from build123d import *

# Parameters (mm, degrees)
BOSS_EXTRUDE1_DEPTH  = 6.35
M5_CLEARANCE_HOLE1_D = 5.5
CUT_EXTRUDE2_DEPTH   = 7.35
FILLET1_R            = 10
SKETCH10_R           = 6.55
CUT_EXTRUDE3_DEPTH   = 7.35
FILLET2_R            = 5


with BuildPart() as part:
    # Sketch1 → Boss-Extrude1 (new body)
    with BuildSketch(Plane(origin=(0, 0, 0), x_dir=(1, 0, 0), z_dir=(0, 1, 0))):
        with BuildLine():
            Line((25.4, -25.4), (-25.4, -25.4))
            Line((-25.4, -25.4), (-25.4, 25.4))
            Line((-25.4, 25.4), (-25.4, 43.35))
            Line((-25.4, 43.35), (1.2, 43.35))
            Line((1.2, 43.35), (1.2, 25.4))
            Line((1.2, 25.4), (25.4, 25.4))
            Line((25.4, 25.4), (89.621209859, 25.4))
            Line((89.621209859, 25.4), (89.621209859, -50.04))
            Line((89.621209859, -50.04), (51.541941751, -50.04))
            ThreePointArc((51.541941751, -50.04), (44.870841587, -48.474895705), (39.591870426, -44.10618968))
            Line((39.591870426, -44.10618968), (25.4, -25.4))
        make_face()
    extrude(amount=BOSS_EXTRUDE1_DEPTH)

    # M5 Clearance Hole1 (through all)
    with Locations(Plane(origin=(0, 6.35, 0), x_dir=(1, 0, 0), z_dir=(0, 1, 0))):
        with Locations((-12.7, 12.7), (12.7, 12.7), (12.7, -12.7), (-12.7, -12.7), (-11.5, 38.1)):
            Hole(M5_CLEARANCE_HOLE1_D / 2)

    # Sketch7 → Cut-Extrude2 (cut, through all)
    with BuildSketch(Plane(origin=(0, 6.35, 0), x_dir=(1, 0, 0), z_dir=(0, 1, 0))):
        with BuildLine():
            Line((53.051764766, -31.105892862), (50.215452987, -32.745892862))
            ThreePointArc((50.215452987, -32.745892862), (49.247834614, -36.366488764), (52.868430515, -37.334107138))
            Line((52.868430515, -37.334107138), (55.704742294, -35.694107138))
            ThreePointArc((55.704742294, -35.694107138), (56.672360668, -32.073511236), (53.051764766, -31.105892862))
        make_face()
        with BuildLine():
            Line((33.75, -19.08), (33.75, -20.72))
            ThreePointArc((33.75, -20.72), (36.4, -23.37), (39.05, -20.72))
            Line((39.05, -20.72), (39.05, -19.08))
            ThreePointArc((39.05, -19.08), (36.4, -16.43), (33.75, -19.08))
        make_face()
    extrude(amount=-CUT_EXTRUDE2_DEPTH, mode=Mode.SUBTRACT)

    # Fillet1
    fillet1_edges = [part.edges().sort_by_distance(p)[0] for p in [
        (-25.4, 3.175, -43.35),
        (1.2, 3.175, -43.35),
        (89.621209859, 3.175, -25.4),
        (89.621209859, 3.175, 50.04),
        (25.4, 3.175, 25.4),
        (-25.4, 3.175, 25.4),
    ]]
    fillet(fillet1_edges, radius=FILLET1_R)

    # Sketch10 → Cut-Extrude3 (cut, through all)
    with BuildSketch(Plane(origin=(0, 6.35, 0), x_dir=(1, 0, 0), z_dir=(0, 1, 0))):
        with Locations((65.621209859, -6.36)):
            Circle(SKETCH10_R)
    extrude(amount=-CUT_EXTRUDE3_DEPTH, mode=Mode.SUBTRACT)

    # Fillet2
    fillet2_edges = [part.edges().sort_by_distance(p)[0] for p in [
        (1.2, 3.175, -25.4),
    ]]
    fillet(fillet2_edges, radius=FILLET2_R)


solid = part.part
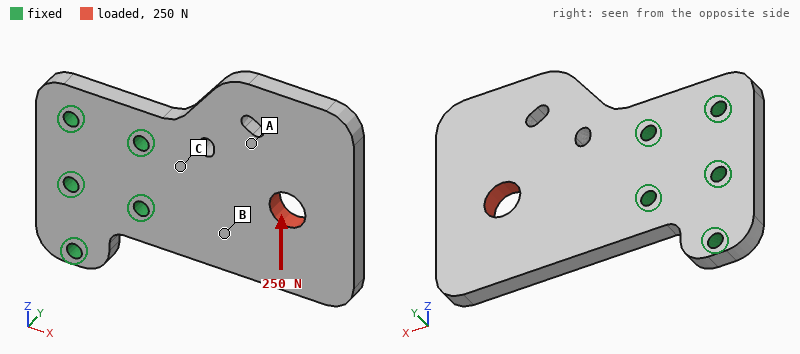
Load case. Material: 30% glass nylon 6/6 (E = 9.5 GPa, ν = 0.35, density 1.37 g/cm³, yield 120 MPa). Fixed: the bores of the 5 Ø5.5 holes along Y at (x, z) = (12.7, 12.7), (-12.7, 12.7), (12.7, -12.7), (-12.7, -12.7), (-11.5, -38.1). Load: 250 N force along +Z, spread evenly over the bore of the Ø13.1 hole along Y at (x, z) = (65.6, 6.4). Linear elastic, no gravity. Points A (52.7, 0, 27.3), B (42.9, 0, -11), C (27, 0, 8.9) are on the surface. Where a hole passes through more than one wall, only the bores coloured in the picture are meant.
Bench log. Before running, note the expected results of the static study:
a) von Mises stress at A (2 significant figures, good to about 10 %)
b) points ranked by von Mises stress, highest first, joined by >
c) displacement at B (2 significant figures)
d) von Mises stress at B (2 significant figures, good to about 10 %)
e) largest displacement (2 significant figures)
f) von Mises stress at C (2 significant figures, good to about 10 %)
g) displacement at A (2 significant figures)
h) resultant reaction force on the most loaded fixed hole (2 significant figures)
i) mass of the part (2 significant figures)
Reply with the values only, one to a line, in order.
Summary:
0.78 MPa
C > B > A
20 µm
1.8 MPa
62 µm
2.7 MPa
33 µm
360 N
63 g
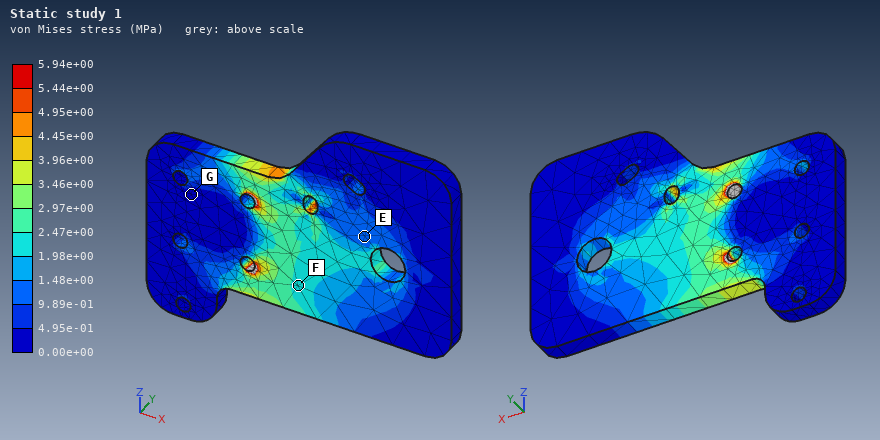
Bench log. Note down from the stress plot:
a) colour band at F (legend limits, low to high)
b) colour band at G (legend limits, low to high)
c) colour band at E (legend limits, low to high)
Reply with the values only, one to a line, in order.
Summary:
1.98e+00 to 2.47e+00 MPa
0.00e+00 to 4.95e-01 MPa
9.89e-01 to 1.48e+00 MPa
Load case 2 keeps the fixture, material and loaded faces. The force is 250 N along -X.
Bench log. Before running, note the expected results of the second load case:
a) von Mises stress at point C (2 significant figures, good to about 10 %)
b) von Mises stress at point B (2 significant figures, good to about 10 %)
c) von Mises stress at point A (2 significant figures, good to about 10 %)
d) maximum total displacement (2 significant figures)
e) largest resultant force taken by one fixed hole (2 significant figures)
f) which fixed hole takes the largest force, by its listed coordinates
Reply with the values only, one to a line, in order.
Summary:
1.1 MPa
0.62 MPa
0.48 MPa
8.9 µm
150 N
(12.7, 12.7)
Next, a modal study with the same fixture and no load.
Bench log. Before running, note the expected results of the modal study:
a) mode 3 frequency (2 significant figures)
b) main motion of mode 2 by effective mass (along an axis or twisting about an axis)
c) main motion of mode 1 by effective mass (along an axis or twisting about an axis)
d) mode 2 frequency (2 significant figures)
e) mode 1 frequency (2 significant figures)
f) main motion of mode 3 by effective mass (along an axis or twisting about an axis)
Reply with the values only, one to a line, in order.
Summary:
2100 Hz
twisting about X
along Y
890 Hz
390 Hz
along Z
